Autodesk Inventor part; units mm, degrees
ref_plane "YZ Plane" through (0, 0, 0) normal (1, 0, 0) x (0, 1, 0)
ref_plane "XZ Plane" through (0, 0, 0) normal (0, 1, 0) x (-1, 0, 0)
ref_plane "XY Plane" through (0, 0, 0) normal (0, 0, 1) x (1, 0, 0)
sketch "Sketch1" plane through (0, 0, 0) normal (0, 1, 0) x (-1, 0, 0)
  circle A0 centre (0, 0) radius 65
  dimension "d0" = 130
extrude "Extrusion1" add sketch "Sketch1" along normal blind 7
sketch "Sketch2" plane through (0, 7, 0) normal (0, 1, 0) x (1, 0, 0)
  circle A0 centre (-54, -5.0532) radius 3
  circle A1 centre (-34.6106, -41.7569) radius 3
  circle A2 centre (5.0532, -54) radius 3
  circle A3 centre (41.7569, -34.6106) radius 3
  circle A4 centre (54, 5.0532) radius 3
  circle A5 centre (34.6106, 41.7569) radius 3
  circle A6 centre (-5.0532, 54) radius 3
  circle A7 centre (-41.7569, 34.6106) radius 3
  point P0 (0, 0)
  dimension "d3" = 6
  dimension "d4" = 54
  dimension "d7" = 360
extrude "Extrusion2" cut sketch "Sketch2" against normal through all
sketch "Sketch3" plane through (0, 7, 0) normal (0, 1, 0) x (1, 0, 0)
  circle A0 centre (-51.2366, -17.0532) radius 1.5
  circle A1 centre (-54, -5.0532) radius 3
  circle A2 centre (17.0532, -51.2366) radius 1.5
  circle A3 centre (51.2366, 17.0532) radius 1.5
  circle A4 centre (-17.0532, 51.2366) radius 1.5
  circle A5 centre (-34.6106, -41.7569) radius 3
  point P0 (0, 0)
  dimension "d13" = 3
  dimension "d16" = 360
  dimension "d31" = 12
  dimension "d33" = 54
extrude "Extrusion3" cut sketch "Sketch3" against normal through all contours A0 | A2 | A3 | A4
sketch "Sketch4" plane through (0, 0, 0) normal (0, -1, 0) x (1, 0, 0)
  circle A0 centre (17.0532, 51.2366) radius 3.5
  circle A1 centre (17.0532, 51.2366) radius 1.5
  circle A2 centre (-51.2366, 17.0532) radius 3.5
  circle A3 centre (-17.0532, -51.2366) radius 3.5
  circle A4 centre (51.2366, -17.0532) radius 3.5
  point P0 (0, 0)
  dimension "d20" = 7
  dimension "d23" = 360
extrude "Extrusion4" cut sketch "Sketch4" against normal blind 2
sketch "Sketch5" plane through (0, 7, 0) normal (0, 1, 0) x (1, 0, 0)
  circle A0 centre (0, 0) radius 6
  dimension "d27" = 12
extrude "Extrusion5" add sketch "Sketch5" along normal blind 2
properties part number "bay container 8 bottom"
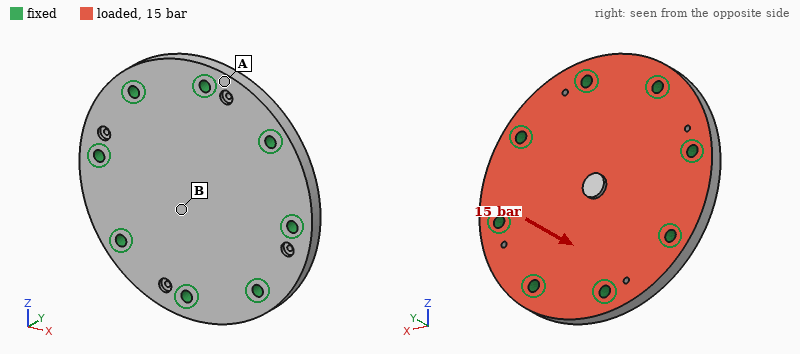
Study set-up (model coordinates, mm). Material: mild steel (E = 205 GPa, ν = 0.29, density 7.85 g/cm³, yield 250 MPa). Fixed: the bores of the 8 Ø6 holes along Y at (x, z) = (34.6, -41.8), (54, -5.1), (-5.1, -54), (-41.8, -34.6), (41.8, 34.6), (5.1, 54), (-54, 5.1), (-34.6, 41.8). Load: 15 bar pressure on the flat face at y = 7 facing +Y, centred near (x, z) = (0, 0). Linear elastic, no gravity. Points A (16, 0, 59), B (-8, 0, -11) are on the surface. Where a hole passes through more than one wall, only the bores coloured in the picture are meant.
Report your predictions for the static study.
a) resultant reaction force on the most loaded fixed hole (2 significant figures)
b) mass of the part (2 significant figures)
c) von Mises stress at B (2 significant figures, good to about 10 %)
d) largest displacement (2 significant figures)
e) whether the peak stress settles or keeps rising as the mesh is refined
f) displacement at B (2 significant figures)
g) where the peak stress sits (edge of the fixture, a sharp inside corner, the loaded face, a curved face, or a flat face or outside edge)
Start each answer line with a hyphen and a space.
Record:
- 2.4 kN
- 720 g
- 39 MPa
- 37 µm
- keeps rising
- 33 µm
- edge of the fixture
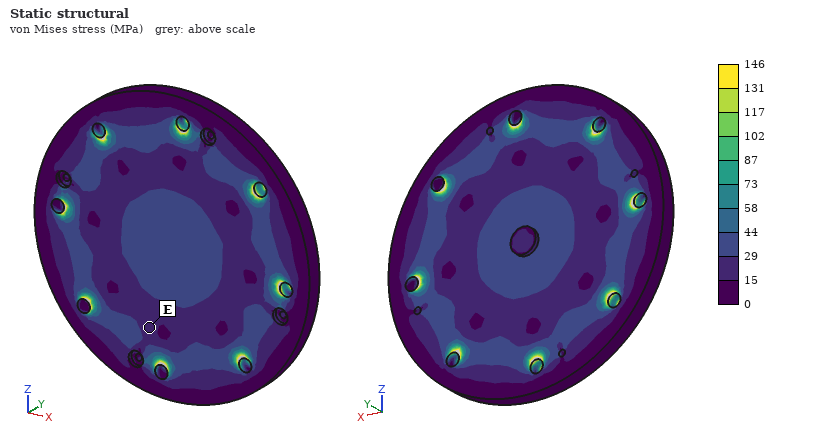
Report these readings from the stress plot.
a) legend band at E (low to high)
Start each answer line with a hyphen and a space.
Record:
- 15 to 29 MPa
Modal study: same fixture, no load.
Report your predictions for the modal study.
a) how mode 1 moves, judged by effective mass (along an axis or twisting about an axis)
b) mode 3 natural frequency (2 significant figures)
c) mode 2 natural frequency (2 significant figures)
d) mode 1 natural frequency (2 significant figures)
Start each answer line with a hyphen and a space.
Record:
- along Y
- 10 kHz
- 10 kHz
- 5200 Hz
